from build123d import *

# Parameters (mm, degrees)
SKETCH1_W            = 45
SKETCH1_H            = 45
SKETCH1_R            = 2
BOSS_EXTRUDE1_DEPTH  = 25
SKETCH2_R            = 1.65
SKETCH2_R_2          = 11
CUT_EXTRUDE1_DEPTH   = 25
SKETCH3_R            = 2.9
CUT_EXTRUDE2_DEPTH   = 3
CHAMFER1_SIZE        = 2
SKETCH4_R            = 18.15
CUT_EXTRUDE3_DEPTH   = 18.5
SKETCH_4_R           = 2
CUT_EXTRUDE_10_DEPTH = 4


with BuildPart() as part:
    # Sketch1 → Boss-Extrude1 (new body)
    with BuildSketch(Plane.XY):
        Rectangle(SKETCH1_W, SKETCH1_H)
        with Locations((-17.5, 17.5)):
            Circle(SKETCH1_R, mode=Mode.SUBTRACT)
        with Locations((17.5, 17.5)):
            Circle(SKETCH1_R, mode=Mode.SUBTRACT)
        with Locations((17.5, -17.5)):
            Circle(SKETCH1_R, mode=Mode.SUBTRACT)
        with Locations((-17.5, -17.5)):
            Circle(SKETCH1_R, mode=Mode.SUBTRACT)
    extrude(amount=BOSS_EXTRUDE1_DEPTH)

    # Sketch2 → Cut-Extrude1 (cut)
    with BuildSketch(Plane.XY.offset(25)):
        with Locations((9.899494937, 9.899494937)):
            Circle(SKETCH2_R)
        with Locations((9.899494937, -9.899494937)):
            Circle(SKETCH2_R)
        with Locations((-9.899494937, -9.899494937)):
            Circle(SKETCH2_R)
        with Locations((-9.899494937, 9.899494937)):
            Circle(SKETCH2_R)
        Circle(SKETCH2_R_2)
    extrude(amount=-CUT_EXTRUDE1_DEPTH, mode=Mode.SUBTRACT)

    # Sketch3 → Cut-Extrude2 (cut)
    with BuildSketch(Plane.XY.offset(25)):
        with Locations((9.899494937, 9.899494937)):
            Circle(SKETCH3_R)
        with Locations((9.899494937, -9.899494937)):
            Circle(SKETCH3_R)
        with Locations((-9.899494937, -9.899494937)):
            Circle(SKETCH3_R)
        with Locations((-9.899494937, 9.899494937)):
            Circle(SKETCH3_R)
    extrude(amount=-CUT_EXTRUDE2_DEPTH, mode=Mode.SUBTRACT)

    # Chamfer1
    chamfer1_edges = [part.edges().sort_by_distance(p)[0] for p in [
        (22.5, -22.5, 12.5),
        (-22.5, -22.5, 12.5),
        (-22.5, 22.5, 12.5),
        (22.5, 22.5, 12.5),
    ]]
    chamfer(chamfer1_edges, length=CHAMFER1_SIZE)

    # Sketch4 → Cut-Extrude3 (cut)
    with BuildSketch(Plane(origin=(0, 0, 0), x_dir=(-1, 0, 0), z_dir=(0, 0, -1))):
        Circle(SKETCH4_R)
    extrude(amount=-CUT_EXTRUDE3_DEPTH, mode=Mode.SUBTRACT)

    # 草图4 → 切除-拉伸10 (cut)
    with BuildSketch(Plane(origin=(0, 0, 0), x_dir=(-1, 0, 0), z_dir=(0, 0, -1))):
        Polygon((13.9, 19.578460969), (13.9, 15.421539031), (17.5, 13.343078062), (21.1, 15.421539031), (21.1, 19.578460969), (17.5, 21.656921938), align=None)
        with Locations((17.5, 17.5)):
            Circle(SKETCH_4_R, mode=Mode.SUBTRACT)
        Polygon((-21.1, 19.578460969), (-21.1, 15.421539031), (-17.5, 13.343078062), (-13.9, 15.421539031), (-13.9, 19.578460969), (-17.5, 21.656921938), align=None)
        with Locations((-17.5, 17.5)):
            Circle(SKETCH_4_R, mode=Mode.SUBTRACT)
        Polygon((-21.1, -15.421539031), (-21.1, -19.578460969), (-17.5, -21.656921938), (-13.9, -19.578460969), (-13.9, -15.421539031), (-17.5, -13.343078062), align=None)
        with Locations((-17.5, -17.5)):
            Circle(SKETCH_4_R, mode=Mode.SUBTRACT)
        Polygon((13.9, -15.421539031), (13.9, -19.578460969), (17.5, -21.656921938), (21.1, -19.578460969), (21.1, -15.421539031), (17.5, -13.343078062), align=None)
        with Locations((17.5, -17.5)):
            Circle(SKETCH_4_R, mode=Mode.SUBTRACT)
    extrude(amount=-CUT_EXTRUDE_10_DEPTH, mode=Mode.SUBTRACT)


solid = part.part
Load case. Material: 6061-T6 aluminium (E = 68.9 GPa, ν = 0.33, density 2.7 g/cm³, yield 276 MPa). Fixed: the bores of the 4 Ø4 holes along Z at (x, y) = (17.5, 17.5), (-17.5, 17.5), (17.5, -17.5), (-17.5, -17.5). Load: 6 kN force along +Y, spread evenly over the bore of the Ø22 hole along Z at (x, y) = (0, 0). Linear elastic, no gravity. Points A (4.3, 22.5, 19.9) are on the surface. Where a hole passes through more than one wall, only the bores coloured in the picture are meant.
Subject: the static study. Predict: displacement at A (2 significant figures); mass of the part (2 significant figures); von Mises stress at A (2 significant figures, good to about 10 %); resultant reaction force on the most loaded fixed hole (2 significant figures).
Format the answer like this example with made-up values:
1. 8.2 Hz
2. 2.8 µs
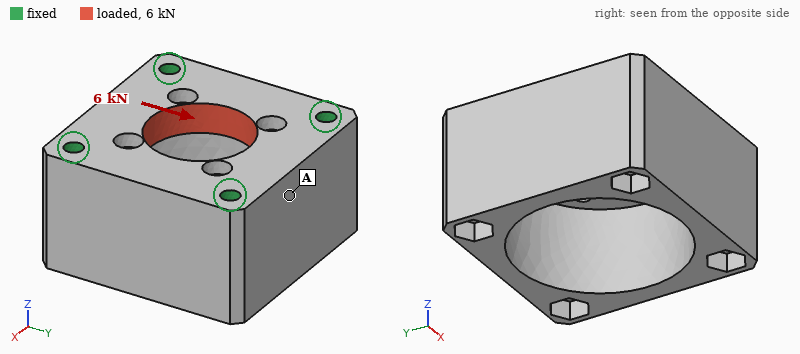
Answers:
1. 5.2 µm
2. 72 g
3. 14 MPa
4. 1.6 kN
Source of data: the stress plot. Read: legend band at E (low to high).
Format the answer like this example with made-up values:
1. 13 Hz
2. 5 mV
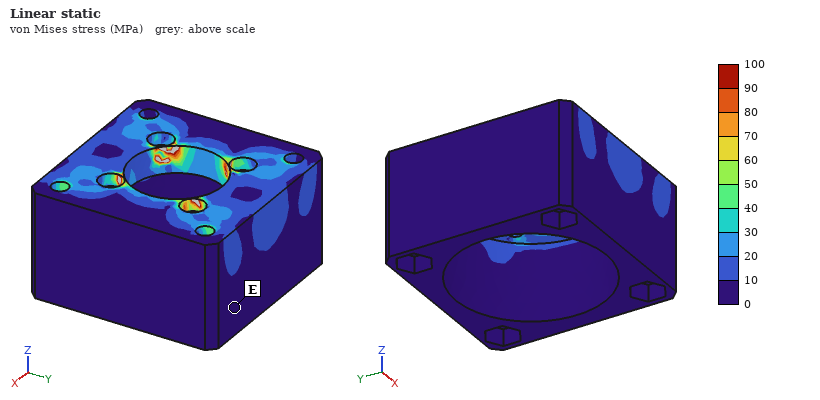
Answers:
1. 0 to 10 MPa
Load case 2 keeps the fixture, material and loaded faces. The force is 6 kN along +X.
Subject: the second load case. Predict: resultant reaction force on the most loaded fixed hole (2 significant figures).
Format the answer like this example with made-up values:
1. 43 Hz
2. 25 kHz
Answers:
1. 1.6 kN
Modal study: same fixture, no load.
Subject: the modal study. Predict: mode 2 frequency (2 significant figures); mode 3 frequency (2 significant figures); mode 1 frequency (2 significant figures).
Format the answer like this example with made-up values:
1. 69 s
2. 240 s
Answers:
1. 32 kHz
2. 32 kHz
3. 25 kHz
